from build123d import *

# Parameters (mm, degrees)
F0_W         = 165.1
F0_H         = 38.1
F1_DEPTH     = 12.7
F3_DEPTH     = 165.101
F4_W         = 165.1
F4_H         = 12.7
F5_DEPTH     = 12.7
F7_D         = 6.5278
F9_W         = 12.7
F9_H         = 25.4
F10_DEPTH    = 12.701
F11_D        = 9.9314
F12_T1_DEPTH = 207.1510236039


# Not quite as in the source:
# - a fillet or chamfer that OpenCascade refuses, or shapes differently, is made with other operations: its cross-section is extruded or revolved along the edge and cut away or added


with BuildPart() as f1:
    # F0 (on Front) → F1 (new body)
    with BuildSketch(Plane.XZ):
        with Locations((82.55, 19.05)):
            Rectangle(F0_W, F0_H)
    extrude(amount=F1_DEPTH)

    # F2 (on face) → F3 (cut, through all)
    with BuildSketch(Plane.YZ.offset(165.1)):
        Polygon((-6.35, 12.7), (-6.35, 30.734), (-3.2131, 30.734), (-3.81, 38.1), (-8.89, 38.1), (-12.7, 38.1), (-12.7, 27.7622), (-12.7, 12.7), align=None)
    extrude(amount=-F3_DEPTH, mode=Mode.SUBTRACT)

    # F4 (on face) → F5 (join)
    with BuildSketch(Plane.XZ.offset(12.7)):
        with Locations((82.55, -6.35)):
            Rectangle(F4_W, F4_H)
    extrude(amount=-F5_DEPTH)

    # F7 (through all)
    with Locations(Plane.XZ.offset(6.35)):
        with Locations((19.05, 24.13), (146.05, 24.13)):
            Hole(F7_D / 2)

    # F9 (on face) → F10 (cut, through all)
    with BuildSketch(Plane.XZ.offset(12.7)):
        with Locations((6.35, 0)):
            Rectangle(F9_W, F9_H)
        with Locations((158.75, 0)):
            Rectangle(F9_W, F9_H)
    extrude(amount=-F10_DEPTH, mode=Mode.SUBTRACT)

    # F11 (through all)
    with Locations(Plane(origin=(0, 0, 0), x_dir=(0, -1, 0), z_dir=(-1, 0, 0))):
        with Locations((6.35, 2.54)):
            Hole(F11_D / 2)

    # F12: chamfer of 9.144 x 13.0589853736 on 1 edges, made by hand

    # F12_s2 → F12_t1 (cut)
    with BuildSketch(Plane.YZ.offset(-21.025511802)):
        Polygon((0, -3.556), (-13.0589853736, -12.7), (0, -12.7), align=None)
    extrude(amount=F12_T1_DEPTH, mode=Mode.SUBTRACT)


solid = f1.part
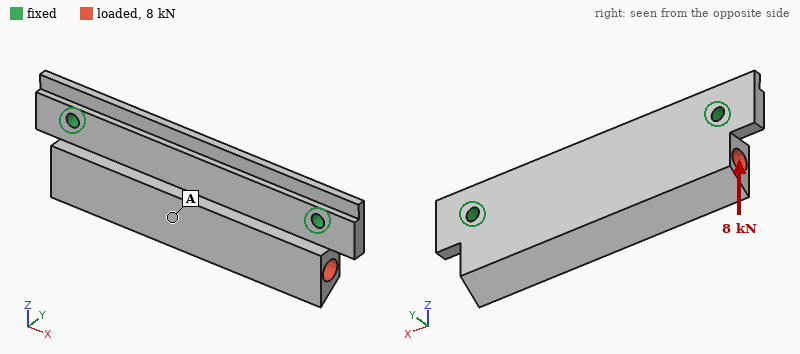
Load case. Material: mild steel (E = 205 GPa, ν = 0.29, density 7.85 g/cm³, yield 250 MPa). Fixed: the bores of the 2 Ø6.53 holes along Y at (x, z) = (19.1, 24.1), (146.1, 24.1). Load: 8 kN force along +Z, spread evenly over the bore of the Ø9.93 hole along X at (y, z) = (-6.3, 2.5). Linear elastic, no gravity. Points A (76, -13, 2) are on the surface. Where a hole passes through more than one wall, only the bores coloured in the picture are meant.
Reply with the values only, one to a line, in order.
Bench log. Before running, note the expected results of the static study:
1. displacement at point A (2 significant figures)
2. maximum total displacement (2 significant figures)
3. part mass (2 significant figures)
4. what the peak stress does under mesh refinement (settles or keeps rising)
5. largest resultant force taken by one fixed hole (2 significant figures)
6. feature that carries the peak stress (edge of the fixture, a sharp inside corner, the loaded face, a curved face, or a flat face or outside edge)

56 µm
77 µm
380 g
keeps rising
4.5 kN
edge of the fixture
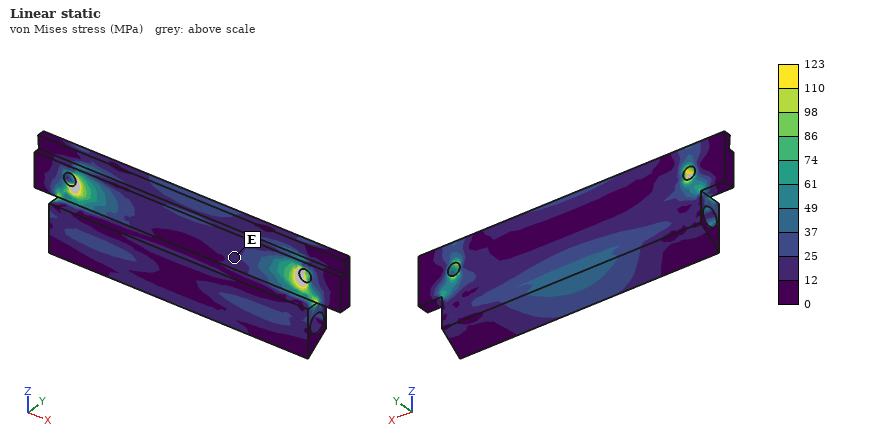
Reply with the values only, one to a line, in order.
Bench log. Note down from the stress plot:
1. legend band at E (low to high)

12 to 25 MPa
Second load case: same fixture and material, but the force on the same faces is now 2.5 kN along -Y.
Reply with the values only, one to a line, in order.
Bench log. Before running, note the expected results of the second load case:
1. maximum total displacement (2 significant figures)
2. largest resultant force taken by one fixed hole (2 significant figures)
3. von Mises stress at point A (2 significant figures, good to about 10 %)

0.12 mm
1.3 kN
37 MPa
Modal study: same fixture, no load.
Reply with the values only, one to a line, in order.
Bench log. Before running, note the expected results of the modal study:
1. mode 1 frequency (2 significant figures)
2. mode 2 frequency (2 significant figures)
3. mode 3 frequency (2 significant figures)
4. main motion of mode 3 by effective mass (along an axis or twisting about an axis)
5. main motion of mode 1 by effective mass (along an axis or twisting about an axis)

1900 Hz
3100 Hz
4900 Hz
twisting about Z
along Y
